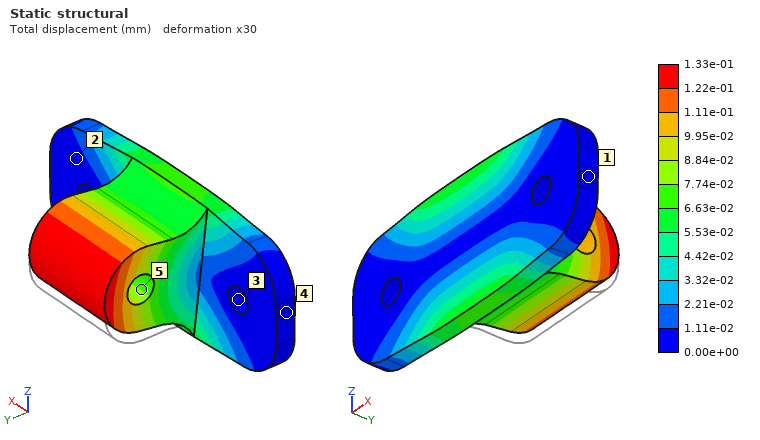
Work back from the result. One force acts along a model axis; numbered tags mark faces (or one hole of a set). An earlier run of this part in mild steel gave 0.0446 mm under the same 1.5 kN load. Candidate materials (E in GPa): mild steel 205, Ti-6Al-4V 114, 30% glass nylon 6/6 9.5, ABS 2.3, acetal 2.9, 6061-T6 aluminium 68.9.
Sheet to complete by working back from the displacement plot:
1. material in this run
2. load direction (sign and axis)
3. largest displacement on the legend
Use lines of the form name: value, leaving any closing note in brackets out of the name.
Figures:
material in this run: 6061-T6 aluminium
load direction: +Z
largest displacement on the legend: 1.33e-01 mm
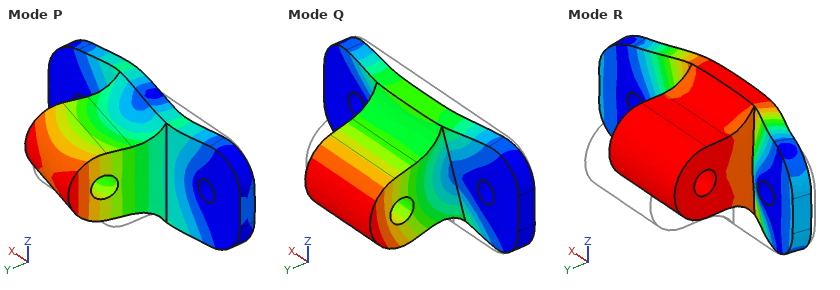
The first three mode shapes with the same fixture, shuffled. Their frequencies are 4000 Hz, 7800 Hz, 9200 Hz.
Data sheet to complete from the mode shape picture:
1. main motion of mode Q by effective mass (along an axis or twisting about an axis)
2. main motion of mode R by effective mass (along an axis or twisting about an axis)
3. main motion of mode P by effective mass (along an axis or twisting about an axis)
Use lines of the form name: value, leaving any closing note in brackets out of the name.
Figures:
main motion of mode Q by effective mass: along Z
main motion of mode R by effective mass: along Y
main motion of mode P by effective mass: along X
